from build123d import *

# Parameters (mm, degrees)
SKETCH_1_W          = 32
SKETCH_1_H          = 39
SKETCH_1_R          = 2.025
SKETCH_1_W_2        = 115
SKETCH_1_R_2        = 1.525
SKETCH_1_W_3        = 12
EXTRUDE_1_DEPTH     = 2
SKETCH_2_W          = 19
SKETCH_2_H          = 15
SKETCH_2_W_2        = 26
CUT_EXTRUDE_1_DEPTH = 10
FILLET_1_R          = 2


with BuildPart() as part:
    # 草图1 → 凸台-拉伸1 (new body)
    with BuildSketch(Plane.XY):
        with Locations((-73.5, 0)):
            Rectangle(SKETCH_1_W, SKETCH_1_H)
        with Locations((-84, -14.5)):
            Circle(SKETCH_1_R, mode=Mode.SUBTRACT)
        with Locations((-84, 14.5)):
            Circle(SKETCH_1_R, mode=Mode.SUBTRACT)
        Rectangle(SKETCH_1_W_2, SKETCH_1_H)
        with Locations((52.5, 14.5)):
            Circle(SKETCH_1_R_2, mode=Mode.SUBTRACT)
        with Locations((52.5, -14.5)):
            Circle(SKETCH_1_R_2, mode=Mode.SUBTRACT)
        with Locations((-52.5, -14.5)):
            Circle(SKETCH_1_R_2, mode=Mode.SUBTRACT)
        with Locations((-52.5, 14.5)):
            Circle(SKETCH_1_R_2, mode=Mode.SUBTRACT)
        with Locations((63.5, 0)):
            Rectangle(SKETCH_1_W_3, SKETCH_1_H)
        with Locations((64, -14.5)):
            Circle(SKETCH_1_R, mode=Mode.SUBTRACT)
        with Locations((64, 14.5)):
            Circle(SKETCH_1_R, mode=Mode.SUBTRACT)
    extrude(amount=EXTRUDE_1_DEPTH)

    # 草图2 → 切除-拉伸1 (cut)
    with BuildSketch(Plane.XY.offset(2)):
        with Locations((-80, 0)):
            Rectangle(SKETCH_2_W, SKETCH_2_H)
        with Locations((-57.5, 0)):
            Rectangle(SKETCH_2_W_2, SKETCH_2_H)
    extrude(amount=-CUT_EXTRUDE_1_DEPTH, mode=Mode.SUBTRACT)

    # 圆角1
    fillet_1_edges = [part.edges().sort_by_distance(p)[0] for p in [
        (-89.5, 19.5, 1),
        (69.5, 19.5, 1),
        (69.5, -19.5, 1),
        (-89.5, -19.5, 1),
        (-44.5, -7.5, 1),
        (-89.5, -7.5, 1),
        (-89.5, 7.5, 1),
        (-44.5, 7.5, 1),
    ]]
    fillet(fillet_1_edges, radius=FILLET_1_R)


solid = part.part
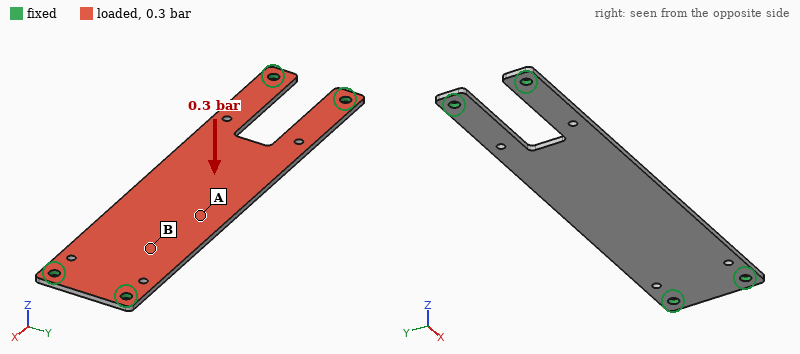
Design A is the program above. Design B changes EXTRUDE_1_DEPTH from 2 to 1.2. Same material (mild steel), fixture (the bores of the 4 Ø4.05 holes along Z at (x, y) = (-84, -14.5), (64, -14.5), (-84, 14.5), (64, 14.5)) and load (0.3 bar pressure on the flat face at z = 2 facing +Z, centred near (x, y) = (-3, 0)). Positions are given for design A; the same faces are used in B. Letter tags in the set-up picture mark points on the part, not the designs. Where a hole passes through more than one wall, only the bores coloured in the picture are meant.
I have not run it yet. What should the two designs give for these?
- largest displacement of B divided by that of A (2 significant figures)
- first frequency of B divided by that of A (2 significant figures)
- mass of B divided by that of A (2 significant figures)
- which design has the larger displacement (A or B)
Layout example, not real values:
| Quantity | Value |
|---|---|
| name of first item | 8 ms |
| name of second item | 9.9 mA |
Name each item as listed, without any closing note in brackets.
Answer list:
| Quantity | Value |
|---|---|
| largest displacement of B divided by that of A | 4.6 |
| first frequency of B divided by that of A | 0.60 |
| mass of B divided by that of A | 0.60 |
| which design has the larger displacement | B |
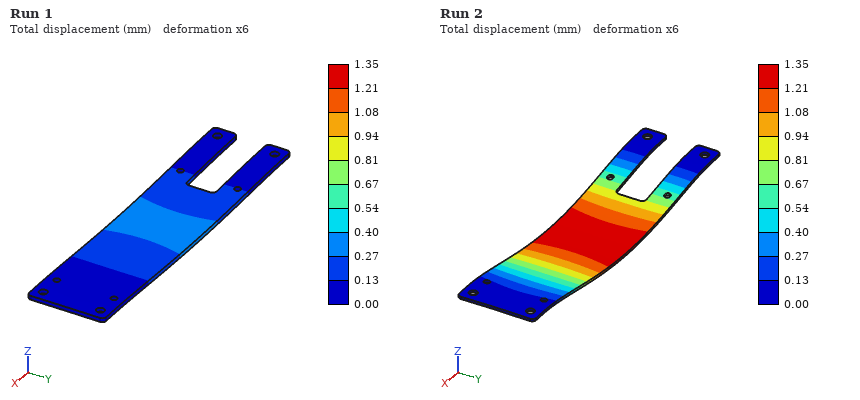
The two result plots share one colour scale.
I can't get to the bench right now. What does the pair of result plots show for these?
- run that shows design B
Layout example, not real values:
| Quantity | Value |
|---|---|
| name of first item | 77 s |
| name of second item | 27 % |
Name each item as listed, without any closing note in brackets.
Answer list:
| Quantity | Value |
|---|---|
| run that shows design B | Run 2 |
